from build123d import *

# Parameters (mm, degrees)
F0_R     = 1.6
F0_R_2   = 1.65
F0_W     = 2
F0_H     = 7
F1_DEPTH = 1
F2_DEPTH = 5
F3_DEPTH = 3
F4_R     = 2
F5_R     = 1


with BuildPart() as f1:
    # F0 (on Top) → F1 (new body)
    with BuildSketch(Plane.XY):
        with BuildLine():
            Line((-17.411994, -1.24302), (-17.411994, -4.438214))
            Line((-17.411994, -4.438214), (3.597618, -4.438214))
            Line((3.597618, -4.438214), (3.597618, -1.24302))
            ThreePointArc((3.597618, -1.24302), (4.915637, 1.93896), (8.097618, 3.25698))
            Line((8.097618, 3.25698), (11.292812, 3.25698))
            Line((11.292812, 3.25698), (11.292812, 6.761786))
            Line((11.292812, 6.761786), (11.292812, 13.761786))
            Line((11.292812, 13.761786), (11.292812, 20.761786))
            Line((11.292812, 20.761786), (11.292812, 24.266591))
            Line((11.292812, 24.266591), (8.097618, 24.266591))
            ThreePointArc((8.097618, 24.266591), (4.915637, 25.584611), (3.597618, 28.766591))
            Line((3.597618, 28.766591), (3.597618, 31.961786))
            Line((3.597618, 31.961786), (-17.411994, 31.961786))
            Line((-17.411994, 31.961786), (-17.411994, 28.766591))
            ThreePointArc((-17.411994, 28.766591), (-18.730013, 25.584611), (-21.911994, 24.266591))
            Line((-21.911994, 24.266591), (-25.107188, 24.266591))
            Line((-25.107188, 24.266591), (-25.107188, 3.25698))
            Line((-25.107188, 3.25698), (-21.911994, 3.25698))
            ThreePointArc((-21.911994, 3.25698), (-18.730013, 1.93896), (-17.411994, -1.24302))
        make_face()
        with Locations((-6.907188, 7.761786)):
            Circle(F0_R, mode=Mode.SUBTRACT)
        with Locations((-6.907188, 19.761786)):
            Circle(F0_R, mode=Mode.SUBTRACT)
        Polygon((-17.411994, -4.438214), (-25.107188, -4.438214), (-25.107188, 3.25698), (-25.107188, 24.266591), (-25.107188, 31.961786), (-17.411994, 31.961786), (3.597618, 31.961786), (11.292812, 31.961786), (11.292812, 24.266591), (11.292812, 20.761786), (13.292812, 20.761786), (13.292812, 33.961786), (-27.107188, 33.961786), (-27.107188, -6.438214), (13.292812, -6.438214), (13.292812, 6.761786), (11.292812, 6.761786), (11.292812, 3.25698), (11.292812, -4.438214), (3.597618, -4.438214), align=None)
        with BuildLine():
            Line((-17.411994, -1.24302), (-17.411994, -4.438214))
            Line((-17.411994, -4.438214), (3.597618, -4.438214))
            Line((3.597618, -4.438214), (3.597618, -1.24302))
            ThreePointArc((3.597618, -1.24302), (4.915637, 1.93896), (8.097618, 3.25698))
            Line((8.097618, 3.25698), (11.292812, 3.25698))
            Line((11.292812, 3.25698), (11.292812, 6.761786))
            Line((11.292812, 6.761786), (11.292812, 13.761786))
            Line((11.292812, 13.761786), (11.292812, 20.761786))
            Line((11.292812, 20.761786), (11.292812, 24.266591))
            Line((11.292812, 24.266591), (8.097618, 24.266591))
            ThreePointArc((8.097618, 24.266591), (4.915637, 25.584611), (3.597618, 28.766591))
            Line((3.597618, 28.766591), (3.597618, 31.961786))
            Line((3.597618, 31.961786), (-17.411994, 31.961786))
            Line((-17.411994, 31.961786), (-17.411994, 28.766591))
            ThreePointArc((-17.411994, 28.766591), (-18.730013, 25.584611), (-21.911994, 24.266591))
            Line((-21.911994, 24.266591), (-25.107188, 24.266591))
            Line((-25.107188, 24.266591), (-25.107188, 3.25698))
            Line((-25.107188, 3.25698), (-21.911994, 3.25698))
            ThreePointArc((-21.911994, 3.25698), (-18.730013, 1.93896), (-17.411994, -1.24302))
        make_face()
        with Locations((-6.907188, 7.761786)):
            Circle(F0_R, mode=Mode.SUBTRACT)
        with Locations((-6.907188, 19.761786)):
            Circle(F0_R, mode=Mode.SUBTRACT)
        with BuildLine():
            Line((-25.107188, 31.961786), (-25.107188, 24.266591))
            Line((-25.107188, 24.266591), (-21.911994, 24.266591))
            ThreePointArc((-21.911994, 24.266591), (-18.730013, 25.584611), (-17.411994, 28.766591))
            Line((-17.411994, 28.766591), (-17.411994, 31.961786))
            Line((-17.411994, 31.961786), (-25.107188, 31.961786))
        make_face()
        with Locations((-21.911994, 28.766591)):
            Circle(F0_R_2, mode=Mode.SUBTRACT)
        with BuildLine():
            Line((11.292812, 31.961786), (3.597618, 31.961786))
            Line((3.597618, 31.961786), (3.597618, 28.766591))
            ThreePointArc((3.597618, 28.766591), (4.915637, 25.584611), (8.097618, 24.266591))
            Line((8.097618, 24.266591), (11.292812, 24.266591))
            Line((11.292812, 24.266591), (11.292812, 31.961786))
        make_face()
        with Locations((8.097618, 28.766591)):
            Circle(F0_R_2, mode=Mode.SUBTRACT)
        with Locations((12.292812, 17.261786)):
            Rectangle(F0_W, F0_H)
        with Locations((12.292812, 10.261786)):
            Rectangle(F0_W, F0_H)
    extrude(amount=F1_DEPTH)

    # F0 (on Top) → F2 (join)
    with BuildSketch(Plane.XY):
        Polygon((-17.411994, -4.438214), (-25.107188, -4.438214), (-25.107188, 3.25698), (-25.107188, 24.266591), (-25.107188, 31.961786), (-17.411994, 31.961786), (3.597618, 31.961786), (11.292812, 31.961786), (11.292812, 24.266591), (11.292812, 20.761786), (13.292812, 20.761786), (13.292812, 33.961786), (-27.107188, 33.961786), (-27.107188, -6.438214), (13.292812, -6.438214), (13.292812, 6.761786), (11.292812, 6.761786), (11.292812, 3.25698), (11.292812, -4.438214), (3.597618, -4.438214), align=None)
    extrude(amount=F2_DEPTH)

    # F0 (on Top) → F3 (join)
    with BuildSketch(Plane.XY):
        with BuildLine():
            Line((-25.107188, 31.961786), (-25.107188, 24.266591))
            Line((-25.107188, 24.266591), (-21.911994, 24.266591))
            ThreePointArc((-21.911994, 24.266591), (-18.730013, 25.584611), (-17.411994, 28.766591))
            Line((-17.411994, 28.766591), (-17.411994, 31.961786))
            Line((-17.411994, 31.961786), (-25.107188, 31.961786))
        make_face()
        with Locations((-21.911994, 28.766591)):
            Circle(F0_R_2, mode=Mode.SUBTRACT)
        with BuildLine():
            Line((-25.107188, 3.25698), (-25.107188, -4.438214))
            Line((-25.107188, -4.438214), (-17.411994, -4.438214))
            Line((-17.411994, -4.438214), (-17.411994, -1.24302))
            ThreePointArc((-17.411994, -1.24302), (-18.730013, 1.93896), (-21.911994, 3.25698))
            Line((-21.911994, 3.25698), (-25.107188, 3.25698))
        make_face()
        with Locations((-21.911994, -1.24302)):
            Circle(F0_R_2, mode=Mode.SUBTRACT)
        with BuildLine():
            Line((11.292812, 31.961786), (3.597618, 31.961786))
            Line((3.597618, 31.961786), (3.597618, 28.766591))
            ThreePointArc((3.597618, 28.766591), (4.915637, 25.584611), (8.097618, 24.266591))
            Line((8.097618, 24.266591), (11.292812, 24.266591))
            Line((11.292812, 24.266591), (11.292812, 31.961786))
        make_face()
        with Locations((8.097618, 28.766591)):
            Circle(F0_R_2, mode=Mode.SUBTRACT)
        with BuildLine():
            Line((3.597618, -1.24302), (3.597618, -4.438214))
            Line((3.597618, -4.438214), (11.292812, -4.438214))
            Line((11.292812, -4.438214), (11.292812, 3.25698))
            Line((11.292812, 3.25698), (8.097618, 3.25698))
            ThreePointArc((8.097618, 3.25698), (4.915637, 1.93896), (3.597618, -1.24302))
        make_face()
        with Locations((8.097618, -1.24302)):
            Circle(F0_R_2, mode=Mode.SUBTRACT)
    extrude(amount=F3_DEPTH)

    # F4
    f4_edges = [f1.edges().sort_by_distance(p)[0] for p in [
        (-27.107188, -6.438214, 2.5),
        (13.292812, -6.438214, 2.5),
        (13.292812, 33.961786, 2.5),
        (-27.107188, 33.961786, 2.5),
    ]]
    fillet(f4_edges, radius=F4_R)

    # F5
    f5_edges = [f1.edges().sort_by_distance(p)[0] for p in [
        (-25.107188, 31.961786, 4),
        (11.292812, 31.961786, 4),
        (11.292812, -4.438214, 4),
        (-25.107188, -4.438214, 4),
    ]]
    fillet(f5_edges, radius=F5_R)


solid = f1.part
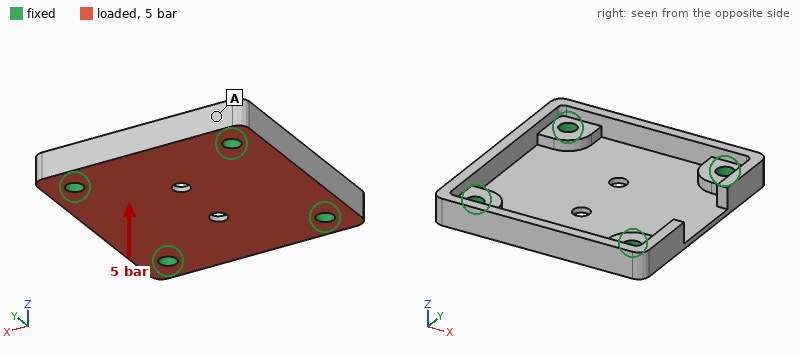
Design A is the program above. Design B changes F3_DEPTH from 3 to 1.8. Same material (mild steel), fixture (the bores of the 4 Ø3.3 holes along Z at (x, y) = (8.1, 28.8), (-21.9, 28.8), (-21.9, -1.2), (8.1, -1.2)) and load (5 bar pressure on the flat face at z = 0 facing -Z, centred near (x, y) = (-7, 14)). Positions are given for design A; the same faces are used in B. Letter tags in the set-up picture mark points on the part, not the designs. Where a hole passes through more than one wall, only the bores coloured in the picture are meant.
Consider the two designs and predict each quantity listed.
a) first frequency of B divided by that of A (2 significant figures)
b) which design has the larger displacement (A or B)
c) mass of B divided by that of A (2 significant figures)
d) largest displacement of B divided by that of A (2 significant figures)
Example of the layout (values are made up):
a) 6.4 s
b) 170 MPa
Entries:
a) 0.95
b) B
c) 0.93
d) 1.1
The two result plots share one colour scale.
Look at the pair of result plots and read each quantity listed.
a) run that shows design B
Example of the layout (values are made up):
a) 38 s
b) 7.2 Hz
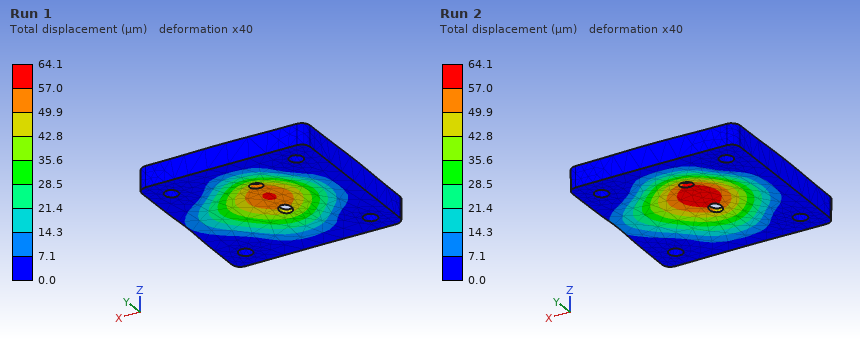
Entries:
a) Run 2
